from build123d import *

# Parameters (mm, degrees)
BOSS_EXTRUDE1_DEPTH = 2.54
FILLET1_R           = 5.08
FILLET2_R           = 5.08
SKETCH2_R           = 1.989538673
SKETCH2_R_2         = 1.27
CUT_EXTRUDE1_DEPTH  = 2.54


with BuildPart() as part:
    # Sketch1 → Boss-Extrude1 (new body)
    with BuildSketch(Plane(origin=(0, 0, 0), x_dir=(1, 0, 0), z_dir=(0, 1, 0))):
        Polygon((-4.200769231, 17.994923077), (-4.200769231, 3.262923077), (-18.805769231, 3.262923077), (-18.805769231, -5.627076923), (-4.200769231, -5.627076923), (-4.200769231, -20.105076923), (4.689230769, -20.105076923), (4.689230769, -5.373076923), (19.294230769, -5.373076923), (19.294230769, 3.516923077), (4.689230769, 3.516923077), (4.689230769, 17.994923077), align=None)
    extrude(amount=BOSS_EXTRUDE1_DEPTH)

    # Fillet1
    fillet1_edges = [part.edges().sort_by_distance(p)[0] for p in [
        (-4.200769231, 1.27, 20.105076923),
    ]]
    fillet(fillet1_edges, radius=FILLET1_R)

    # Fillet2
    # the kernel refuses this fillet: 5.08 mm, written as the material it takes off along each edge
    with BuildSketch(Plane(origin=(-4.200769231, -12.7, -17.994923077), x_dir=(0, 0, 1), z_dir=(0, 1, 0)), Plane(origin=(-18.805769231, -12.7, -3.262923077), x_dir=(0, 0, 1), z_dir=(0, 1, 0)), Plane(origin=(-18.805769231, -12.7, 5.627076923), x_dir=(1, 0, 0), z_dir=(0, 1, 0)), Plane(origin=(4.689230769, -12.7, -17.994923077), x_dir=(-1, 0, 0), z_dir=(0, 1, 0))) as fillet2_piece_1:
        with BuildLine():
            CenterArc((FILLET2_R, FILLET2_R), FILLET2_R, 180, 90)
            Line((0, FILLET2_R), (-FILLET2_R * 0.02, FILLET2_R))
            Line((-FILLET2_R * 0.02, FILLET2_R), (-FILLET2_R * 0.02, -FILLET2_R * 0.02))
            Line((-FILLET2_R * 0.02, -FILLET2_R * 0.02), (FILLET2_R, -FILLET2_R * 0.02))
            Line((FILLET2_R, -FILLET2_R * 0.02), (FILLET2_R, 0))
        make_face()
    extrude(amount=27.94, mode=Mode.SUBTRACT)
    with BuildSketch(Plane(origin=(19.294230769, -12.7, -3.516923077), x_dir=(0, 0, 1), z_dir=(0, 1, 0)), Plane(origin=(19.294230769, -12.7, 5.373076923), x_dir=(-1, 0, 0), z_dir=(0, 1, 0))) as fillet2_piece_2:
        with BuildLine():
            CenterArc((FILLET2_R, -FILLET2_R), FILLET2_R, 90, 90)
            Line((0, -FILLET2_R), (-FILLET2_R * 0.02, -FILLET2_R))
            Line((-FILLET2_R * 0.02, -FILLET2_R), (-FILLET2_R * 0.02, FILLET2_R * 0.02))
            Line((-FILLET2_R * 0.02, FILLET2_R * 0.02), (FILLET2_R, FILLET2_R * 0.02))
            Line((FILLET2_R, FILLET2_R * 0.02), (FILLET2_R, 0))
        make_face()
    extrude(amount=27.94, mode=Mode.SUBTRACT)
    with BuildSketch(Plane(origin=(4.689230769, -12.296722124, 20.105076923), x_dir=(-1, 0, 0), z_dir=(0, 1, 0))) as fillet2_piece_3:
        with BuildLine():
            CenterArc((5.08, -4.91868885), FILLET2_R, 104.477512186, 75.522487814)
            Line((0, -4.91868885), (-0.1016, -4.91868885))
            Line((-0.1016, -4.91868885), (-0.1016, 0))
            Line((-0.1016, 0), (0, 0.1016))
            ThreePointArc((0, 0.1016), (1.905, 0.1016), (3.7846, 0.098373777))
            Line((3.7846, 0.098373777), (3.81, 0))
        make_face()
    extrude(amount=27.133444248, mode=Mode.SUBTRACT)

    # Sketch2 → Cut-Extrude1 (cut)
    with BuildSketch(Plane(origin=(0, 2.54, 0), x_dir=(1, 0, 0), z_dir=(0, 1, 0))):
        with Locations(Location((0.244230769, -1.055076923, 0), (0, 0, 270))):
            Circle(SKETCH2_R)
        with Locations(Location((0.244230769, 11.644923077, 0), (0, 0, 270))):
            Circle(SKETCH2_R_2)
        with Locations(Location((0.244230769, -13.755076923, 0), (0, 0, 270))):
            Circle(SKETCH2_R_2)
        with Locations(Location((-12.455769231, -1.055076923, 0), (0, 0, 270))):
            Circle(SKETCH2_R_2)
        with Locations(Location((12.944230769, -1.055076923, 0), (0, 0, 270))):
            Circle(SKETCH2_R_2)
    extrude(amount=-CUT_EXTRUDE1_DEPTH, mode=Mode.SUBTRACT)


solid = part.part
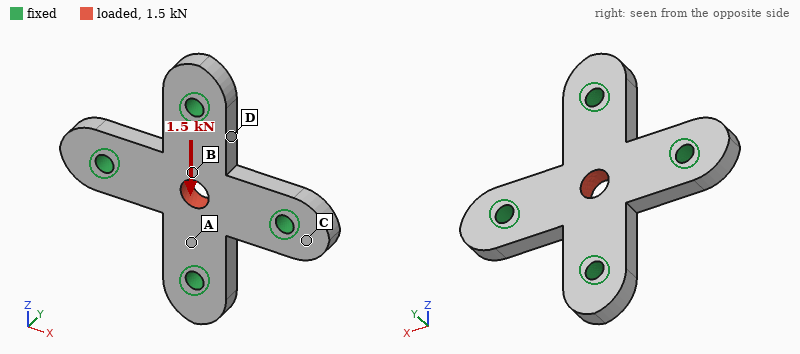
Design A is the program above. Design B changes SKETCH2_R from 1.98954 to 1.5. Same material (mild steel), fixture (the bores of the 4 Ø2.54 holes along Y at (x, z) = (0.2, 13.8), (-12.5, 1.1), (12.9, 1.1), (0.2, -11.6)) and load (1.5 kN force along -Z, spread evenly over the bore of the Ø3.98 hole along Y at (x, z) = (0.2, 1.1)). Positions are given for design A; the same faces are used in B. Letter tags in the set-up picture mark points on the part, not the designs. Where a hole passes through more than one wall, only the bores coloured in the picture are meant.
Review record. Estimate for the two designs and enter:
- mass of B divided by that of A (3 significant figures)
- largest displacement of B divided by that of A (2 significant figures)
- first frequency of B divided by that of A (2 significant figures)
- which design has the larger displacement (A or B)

1.01
1.1
0.99
B
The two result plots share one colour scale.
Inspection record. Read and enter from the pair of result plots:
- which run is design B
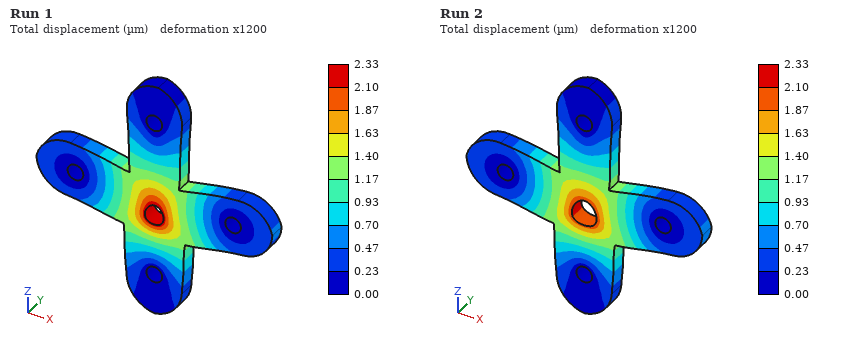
Run 1
